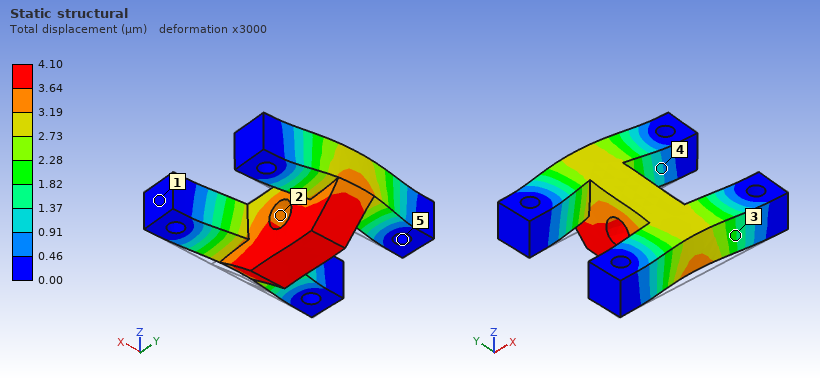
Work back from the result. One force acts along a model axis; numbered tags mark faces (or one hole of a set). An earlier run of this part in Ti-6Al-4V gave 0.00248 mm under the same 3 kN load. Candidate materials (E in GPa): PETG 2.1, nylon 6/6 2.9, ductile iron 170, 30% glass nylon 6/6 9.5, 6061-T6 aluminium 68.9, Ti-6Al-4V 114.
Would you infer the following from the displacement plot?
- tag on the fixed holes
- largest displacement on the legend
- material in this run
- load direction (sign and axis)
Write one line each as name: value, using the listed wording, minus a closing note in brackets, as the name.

tag on the fixed holes: 5
largest displacement on the legend: 4.10 µm
material in this run: 6061-T6 aluminium
load direction: +Y
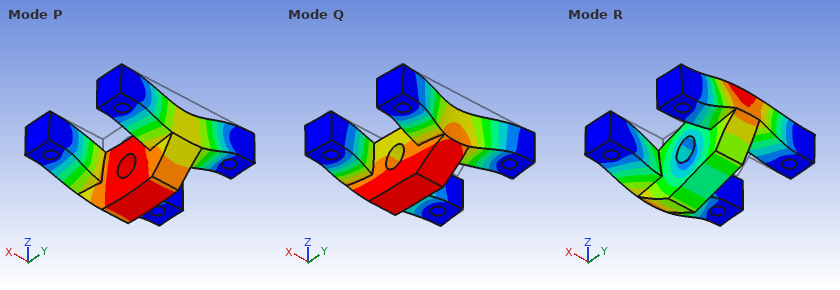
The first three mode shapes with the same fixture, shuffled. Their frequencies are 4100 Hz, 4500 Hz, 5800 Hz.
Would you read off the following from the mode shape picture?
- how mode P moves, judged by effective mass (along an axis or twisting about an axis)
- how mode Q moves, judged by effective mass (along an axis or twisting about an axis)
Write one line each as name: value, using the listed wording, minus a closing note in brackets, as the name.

how mode P moves, judged by effective mass: along Z
how mode Q moves, judged by effective mass: along Y
